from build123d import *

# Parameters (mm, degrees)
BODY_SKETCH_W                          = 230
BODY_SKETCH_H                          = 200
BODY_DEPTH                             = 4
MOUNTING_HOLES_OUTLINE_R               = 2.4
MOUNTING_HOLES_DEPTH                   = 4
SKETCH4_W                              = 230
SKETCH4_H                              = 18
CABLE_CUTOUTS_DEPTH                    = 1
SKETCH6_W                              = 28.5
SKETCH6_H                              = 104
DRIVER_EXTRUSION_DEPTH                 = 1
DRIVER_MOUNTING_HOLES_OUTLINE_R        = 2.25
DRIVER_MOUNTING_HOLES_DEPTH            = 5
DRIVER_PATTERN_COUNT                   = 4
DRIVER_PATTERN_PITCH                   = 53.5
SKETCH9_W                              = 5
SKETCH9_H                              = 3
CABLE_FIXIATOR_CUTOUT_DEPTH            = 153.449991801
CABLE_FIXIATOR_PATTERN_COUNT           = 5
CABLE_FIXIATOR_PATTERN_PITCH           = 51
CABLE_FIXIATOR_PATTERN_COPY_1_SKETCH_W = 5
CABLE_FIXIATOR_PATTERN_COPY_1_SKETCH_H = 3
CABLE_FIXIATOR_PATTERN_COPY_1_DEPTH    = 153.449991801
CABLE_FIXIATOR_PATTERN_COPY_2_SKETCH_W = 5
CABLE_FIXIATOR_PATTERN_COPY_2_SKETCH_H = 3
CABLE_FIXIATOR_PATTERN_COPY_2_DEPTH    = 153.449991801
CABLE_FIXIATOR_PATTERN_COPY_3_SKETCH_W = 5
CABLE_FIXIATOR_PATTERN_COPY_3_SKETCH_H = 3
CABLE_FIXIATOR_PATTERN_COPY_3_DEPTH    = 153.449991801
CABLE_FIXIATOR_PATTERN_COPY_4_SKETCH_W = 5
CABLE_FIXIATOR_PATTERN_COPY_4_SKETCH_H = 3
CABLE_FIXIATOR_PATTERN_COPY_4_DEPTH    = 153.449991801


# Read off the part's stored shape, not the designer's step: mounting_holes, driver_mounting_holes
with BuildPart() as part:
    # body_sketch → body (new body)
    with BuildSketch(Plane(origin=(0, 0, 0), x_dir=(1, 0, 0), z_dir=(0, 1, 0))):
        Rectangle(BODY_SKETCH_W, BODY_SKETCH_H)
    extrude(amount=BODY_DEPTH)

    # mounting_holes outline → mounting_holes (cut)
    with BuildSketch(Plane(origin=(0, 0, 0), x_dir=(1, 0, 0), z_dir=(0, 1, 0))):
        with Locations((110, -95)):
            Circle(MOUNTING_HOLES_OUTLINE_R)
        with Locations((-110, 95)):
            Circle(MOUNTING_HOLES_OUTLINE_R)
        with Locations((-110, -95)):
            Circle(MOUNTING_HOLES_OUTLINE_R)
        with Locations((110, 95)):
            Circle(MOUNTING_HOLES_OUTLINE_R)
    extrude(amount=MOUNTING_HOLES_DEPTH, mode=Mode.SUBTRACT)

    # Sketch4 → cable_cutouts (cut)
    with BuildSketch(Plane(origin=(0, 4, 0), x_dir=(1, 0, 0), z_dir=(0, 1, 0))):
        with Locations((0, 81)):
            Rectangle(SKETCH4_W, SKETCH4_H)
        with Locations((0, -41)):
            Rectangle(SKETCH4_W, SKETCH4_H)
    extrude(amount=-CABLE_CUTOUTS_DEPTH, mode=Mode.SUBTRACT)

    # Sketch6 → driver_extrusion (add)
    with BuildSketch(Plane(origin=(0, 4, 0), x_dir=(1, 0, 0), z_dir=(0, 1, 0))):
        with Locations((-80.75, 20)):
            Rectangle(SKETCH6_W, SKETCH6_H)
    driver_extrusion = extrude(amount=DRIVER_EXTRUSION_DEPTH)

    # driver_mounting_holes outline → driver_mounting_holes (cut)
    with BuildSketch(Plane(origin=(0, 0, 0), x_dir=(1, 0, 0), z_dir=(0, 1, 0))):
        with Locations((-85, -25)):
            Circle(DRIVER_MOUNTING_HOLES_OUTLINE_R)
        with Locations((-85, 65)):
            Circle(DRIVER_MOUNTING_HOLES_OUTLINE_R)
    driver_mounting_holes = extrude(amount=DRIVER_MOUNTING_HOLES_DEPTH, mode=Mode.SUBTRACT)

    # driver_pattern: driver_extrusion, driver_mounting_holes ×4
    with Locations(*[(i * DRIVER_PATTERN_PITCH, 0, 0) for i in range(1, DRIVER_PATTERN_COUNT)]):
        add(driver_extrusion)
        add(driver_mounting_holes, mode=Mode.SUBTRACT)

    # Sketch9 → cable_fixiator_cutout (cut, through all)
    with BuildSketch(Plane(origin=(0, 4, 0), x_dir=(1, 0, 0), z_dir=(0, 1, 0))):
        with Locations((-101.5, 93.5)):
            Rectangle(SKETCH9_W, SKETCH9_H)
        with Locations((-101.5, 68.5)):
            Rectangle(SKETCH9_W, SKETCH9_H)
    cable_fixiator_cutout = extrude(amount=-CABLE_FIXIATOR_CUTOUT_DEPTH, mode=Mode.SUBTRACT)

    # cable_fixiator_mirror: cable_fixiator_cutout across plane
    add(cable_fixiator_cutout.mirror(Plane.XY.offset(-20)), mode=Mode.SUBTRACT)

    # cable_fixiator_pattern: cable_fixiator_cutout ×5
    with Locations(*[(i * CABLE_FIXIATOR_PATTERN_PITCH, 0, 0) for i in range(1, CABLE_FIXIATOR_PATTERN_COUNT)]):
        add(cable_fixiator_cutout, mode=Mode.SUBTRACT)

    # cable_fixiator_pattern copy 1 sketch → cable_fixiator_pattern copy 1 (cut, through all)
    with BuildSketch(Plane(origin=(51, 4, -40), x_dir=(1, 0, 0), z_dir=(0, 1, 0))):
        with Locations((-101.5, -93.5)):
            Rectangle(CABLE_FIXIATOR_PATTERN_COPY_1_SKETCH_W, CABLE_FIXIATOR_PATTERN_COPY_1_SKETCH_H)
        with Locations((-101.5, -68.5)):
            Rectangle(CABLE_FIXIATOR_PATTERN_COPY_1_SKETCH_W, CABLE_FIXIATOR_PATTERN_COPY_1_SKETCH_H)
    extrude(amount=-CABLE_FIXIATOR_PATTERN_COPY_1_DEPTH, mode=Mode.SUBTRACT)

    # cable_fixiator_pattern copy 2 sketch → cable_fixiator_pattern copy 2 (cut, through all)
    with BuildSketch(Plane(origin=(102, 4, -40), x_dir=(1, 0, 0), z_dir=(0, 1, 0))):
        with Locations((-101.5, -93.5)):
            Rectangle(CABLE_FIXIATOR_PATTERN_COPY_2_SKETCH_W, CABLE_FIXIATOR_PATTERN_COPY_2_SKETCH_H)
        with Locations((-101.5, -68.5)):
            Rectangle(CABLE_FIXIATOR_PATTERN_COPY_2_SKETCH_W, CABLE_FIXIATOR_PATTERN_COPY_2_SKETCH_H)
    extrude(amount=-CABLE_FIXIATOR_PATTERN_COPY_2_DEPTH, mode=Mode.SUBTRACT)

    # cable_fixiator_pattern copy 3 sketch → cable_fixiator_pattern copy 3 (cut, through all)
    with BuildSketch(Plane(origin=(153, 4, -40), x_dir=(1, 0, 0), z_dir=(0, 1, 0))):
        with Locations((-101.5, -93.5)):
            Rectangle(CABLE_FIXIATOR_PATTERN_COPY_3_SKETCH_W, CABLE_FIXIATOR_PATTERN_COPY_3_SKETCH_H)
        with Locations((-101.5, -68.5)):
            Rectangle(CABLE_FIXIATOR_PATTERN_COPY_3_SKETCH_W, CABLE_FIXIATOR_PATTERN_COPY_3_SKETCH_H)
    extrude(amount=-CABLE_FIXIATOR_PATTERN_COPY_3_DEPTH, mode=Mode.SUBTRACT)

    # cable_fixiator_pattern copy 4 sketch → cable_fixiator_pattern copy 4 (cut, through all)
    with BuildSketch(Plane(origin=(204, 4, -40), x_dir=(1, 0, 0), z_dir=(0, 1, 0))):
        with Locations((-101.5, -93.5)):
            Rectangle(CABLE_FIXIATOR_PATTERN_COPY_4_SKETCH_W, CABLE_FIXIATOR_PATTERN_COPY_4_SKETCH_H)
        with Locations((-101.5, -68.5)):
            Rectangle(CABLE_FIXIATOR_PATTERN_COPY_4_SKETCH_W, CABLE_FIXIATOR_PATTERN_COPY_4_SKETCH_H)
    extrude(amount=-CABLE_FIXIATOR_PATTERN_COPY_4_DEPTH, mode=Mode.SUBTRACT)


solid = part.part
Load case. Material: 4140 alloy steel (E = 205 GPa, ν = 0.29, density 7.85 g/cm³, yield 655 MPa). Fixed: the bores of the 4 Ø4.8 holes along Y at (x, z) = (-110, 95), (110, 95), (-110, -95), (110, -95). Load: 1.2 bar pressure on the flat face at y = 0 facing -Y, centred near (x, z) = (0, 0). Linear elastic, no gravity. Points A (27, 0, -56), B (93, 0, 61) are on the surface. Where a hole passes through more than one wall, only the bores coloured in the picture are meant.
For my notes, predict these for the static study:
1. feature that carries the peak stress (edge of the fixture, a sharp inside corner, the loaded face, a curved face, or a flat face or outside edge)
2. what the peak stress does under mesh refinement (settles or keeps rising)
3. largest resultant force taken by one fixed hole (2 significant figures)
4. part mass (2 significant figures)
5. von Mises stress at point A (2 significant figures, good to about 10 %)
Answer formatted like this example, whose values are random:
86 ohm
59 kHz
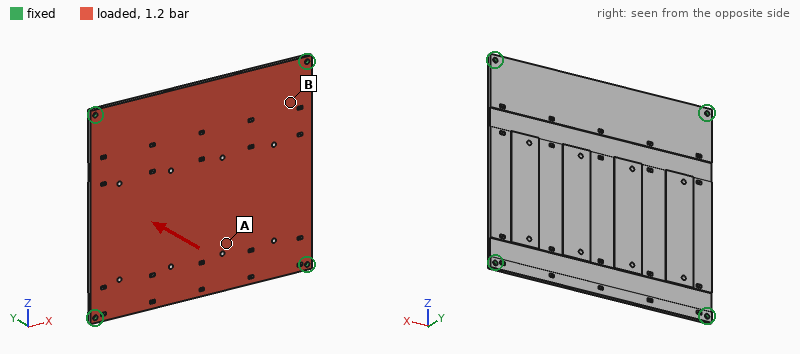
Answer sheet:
edge of the fixture
keeps rising
1.6 kN
1.5 kg
100 MPa
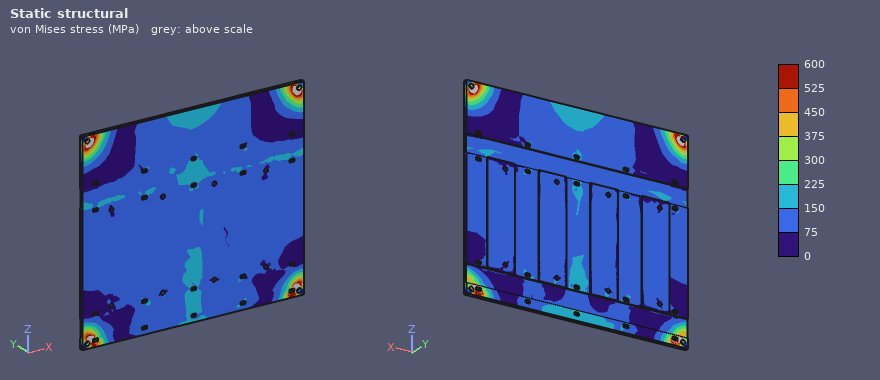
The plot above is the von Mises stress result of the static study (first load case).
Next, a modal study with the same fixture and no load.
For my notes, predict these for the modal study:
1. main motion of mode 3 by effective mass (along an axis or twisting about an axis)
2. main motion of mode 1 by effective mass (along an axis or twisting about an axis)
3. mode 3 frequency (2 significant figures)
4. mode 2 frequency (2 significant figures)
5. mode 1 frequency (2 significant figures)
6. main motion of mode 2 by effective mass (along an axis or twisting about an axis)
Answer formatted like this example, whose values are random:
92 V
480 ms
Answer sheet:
twisting about Z
along Y
530 Hz
480 Hz
260 Hz
twisting about X
